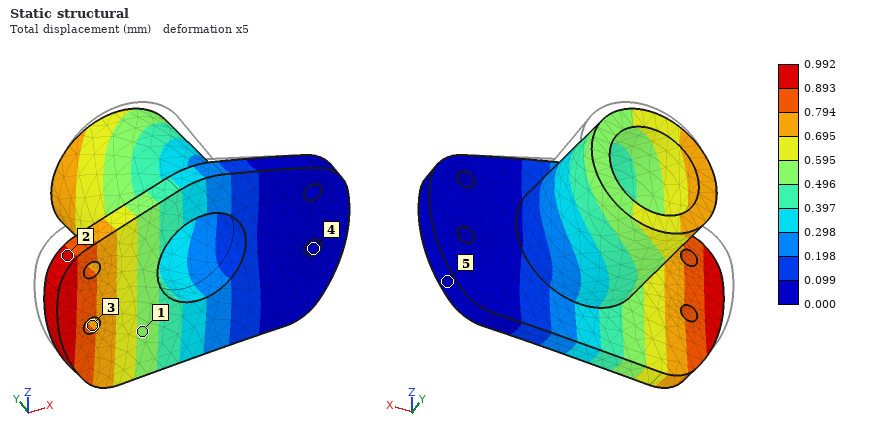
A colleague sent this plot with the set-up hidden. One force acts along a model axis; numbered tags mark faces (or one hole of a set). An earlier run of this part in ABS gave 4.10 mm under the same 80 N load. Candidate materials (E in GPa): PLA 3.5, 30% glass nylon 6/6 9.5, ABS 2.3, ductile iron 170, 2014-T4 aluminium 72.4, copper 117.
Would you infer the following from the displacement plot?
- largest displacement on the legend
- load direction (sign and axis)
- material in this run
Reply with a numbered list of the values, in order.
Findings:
1. 0.992 mm
2. -Y
3. 30% glass nylon 6/6
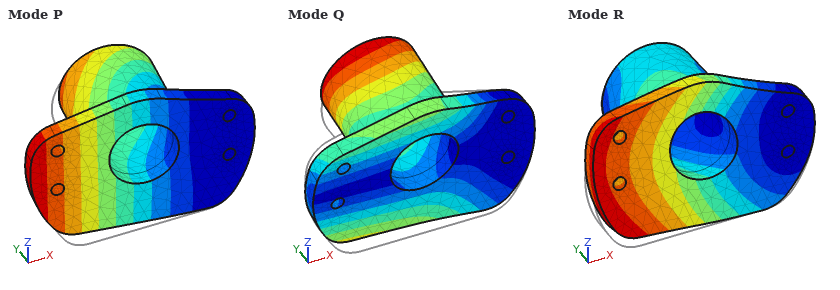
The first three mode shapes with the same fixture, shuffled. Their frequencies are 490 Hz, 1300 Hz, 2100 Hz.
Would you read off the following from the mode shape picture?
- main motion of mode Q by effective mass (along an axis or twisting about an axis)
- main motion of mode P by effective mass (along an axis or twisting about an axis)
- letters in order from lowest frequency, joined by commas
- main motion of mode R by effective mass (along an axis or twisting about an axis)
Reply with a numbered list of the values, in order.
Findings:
1. along Z
2. along Y
3. P, Q, R
4. along Z
